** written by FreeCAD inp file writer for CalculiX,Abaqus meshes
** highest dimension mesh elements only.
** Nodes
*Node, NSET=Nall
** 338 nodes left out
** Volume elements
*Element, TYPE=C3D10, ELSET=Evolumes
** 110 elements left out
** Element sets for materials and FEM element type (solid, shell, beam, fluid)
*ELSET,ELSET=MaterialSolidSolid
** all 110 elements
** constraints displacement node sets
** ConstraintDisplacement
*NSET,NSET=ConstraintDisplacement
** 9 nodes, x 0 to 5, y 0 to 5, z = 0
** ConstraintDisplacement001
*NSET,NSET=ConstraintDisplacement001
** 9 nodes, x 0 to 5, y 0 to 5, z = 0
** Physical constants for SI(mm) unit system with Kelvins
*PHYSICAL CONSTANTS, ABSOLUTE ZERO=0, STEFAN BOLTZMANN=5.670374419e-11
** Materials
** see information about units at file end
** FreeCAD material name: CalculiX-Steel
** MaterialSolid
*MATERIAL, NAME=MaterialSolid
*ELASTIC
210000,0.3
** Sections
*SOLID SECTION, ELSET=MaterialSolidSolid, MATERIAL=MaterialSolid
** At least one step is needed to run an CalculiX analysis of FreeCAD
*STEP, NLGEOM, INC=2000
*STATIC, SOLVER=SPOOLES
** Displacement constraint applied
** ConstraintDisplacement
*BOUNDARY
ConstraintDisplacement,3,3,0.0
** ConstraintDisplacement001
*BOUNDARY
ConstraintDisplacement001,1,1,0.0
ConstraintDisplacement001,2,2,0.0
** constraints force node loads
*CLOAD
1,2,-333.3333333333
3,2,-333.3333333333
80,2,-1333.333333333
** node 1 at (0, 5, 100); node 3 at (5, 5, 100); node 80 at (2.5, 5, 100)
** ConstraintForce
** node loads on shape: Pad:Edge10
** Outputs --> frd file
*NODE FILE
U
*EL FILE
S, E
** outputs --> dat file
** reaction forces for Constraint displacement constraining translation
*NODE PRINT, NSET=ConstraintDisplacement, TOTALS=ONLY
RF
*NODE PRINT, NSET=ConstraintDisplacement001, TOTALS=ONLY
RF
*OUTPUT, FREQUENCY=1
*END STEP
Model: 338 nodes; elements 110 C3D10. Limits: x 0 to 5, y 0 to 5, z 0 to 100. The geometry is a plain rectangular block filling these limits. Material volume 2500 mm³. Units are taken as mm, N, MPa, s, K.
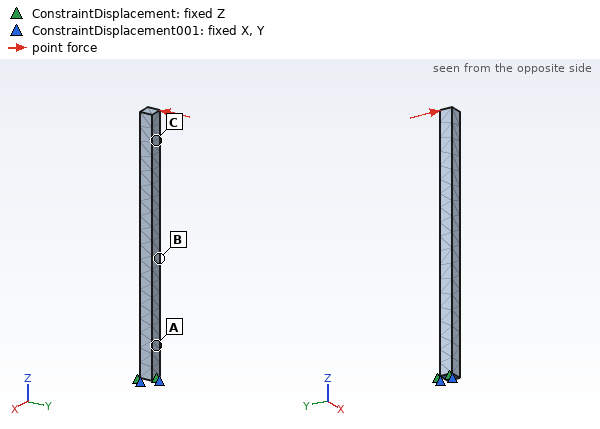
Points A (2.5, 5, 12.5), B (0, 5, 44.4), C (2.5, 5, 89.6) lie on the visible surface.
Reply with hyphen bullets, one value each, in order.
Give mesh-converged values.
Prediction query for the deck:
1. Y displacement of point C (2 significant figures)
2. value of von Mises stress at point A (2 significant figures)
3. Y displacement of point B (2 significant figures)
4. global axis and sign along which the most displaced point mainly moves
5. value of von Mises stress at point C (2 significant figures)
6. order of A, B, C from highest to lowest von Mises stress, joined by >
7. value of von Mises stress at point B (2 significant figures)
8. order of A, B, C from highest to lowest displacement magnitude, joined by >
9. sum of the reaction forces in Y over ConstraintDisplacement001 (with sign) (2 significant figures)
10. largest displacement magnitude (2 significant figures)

- -41 mm
- 7500 MPa
- -13 mm
- -Y
- 940 MPa
- A > B > C
- 4400 MPa
- C > B > A
- 2000 N
- 50 mm
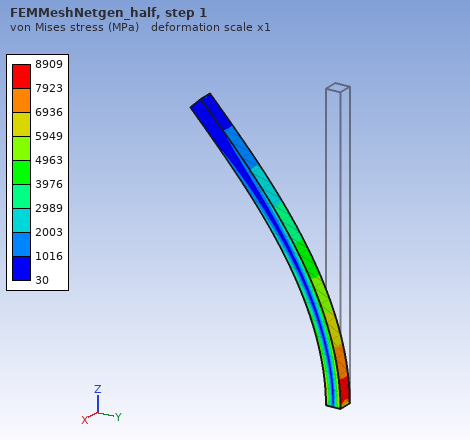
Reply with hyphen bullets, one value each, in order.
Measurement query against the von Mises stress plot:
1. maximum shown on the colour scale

- 8909 MPa
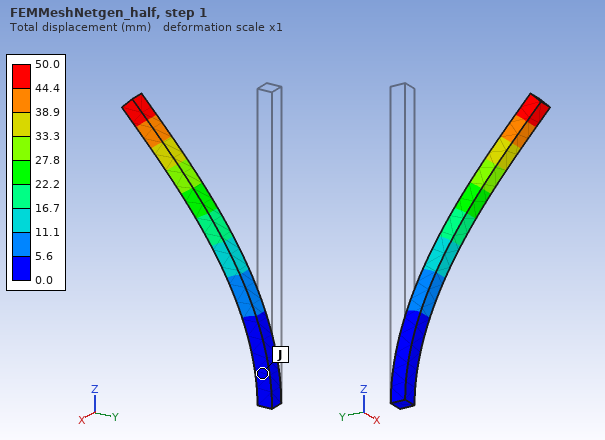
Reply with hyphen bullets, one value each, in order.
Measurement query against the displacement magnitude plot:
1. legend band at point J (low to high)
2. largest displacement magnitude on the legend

- 0.0 to 5.6 mm
- 50.0 mm
